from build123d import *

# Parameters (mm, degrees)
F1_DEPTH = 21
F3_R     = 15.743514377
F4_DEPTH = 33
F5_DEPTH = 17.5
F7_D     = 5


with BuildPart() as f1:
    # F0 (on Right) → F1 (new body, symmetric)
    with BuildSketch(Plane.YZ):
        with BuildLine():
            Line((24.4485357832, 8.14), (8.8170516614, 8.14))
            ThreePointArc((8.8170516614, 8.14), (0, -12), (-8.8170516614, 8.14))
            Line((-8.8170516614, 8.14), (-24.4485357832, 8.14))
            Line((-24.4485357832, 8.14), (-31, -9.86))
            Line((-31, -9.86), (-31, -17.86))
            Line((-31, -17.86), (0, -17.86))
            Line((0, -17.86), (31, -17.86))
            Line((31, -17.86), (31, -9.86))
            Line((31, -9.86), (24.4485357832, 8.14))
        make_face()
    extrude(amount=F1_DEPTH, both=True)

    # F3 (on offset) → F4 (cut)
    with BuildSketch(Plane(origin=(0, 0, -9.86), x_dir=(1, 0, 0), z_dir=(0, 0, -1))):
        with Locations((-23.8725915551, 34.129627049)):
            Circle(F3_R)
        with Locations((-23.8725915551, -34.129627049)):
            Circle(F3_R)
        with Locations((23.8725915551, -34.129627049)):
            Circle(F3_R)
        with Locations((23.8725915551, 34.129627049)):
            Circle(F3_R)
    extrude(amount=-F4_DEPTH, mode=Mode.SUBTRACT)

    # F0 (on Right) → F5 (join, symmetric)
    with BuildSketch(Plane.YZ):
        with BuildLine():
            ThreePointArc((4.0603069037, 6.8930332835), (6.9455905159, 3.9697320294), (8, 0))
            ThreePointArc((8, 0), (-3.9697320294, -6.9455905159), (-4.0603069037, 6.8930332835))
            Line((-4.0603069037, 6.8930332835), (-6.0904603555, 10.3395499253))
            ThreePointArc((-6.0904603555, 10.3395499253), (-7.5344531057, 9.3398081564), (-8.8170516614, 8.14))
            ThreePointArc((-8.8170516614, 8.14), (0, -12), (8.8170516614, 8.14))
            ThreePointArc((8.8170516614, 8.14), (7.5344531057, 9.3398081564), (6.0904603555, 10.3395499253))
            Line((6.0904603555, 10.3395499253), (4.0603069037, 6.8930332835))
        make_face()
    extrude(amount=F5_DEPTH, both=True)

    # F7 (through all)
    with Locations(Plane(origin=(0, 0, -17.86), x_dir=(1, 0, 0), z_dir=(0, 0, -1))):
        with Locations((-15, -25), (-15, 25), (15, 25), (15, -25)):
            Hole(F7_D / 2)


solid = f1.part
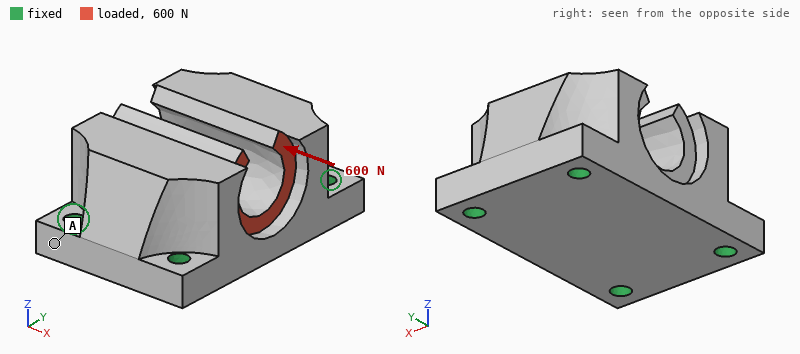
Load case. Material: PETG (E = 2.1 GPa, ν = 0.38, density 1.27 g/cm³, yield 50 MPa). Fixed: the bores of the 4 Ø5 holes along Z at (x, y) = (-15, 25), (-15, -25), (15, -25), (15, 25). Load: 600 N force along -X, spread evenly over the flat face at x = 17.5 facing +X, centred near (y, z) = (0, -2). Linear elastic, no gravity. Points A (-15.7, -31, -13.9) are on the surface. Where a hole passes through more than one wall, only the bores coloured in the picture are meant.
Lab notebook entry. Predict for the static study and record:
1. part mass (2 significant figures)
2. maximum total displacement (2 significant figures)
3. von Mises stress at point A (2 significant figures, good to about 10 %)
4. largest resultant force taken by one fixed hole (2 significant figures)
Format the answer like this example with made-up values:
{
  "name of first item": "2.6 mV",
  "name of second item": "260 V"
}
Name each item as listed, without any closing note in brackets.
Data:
{
  "part mass": "60 g",
  "maximum total displacement": "54 µm",
  "von Mises stress at point A": "0.81 MPa",
  "largest resultant force taken by one fixed hole": "220 N"
}
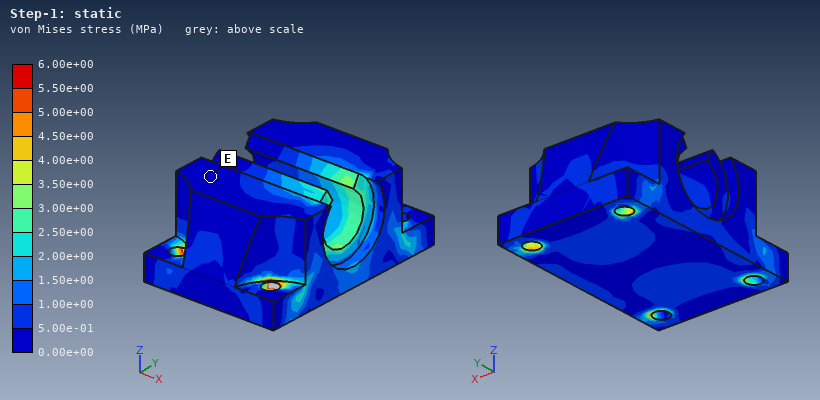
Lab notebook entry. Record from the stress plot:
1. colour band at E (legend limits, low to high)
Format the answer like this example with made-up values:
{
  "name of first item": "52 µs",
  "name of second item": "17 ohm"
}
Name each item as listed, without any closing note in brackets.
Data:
{
  "colour band at E": "0.00e+00 to 5.00e-01 MPa"
}
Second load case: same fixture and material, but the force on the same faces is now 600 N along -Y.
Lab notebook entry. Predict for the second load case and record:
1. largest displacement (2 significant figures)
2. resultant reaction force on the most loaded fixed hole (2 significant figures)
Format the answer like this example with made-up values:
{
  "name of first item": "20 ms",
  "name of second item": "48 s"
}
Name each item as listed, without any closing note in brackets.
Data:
{
  "largest displacement": "78 µm",
  "resultant reaction force on the most loaded fixed hole": "250 N"
}
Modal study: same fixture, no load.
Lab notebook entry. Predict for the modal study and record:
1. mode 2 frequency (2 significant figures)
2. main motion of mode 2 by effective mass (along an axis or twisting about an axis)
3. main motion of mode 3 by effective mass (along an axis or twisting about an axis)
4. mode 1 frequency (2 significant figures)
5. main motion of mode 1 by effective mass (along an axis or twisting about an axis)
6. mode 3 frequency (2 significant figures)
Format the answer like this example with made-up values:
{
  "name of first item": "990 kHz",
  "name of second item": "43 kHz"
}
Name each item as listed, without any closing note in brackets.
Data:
{
  "mode 2 frequency": "4100 Hz",
  "main motion of mode 2 by effective mass": "along X",
  "main motion of mode 3 by effective mass": "along Y",
  "mode 1 frequency": "2400 Hz",
  "main motion of mode 1 by effective mass": "along Z",
  "mode 3 frequency": "4800 Hz"
}
